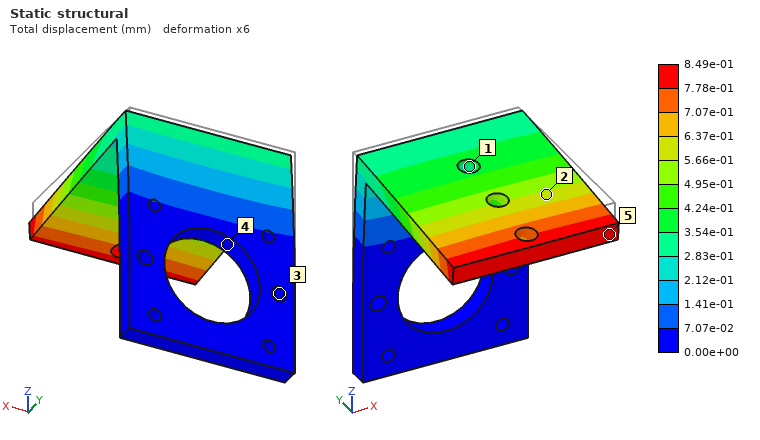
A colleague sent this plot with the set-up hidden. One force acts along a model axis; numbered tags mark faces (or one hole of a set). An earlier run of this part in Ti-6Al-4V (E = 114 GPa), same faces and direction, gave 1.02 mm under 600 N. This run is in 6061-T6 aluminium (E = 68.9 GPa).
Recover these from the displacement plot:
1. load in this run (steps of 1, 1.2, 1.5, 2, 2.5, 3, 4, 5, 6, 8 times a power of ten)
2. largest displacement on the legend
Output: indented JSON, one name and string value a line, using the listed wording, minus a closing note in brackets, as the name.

{
  "load in this run": "300 N",
  "largest displacement on the legend": "8.49e-01 mm"
}
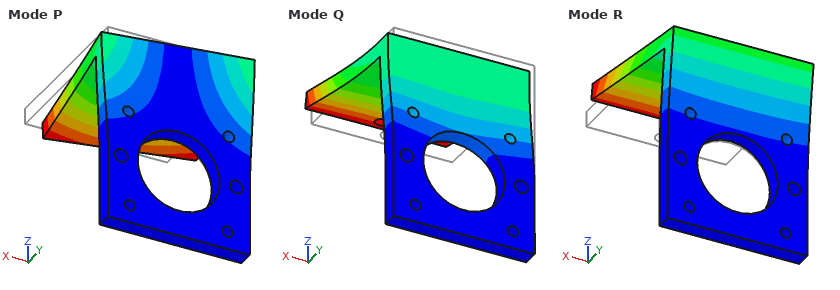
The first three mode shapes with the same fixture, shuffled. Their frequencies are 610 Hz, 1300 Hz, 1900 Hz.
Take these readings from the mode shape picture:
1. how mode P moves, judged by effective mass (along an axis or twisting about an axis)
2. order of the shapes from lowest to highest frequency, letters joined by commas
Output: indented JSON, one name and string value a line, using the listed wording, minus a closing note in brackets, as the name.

{
  "how mode P moves, judged by effective mass": "along X",
  "order of the shapes from lowest to highest frequency, letters joined by commas": "R, P, Q"
}
